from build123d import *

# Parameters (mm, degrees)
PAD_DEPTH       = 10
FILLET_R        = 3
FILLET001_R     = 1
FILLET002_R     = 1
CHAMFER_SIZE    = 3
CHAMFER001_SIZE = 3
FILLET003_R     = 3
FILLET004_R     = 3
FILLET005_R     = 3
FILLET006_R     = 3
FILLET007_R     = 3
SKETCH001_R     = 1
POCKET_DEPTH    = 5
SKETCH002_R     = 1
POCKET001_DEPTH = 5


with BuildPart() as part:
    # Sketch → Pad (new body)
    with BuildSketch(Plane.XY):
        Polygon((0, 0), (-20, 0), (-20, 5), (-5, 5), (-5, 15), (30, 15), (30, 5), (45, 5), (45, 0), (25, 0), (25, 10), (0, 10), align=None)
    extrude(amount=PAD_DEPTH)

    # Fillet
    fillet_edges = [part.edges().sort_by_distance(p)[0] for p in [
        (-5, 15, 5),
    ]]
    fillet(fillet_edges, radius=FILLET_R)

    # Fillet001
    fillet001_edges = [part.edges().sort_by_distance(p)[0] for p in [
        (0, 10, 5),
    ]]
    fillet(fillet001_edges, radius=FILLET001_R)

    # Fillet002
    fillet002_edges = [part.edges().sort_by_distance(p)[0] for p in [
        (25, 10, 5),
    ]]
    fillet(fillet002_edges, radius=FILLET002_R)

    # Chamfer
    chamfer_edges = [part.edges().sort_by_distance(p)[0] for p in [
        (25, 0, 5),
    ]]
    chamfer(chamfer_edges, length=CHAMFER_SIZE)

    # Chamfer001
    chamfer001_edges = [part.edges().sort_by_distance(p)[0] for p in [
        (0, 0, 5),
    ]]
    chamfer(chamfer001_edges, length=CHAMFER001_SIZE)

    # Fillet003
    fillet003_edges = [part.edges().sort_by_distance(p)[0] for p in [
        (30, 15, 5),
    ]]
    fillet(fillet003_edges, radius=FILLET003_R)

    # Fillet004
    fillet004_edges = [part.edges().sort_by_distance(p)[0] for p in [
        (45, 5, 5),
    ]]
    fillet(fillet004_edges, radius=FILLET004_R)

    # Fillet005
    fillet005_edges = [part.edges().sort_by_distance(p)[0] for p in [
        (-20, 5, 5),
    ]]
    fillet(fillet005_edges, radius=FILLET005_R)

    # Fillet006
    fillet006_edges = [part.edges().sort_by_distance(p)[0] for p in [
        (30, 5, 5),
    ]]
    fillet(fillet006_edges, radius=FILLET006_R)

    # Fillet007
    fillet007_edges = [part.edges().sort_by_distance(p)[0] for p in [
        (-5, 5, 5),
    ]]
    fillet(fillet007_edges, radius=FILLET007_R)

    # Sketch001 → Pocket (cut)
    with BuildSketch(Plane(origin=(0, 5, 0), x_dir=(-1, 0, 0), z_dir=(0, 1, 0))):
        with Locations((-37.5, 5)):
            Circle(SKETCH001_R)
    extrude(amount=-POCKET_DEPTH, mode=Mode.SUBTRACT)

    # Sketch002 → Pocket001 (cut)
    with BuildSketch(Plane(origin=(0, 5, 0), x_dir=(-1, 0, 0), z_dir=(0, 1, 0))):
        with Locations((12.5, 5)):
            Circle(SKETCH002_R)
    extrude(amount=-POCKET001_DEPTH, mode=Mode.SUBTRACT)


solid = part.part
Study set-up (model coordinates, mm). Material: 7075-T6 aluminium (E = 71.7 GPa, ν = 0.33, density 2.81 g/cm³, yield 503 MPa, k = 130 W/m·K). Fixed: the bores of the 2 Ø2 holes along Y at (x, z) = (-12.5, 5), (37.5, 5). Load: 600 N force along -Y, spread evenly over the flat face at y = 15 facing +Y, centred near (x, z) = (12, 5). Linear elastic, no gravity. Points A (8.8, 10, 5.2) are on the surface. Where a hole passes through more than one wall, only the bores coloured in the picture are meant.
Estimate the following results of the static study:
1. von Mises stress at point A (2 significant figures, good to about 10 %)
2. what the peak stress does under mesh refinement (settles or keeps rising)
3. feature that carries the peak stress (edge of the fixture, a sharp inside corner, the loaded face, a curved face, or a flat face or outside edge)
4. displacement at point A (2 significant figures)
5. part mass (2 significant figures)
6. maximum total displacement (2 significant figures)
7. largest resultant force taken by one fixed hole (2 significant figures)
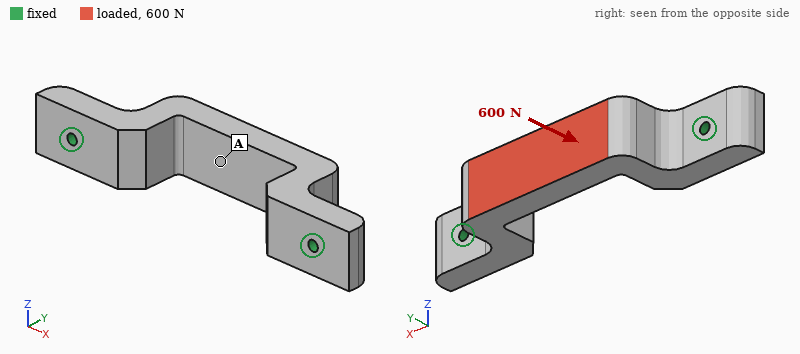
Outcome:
9.5 MPa
keeps rising
edge of the fixture
13 µm
12 g
14 µm
440 N
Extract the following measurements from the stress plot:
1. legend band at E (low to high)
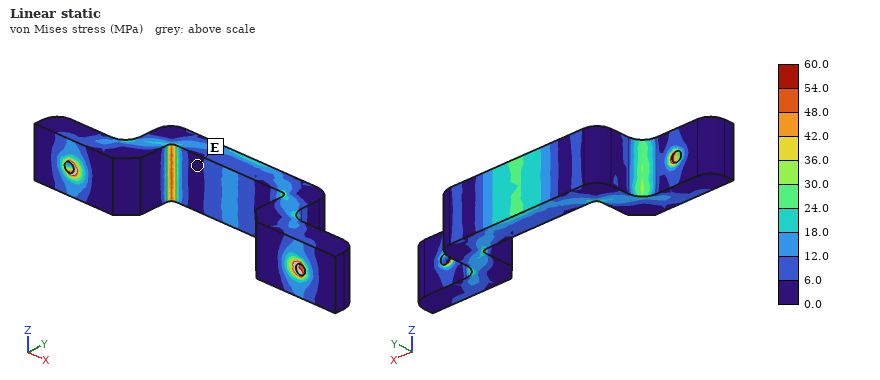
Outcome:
0.0 to 6.0 MPa
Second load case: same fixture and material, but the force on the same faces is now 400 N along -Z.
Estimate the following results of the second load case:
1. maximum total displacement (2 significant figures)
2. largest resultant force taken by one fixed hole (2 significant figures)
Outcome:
58 µm
200 N
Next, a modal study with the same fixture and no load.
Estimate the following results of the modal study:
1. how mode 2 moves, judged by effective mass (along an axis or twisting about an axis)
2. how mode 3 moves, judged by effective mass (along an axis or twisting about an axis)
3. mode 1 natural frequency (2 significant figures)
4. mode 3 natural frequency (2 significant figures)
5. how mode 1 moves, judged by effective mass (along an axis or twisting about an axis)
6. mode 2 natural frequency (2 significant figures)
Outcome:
along X
along Y
6900 Hz
16 kHz
along Z
14 kHz
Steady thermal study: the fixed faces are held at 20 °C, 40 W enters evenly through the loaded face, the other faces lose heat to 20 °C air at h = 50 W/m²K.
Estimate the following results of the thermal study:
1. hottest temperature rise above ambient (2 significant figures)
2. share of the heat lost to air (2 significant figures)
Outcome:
67 K
7.9 %
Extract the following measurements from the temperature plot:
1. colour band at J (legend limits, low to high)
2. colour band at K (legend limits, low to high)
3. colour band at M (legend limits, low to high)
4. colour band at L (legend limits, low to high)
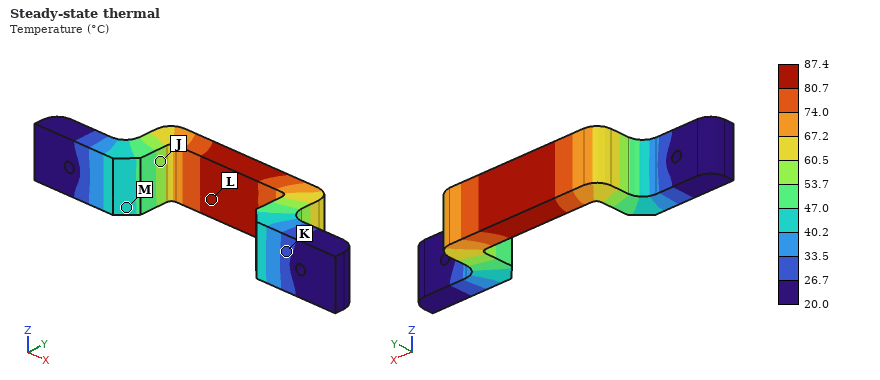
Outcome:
53.7 to 60.5 °C
26.7 to 33.5 °C
40.2 to 47.0 °C
80.7 to 87.4 °C
